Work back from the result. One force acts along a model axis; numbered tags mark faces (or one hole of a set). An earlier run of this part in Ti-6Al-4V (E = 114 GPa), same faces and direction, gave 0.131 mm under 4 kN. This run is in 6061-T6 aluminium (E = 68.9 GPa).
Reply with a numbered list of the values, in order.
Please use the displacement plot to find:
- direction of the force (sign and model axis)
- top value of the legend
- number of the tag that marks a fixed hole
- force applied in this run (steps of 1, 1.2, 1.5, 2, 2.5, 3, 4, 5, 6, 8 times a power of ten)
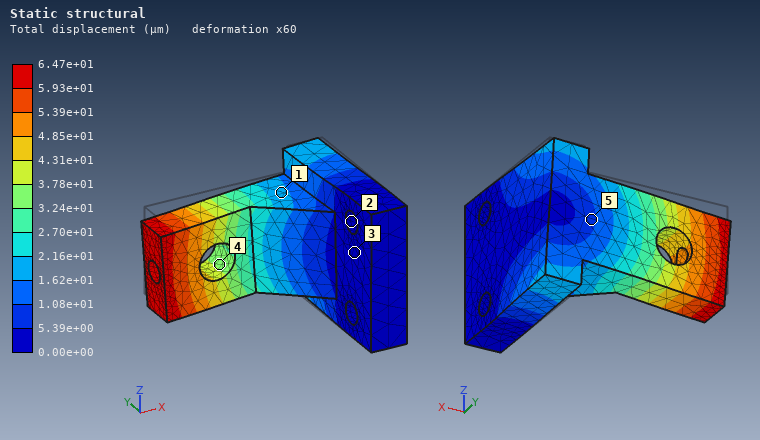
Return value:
1. -Z
2. 6.47e+01 µm
3. 2
4. 1.2 kN
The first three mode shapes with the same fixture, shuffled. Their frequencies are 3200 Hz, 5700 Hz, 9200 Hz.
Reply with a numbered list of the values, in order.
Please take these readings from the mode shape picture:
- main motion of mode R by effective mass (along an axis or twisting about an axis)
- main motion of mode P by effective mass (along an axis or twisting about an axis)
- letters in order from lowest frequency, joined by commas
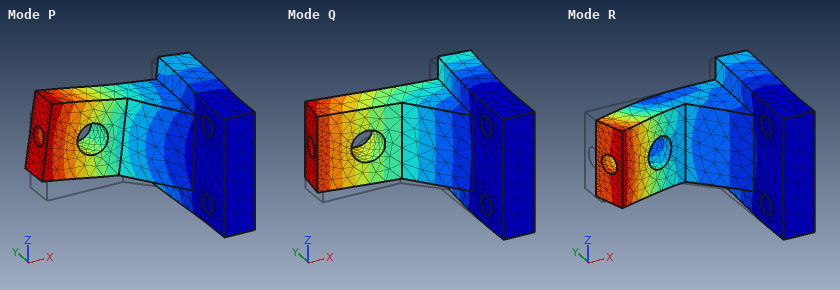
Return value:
1. along X
2. along Z
3. Q, P, R
